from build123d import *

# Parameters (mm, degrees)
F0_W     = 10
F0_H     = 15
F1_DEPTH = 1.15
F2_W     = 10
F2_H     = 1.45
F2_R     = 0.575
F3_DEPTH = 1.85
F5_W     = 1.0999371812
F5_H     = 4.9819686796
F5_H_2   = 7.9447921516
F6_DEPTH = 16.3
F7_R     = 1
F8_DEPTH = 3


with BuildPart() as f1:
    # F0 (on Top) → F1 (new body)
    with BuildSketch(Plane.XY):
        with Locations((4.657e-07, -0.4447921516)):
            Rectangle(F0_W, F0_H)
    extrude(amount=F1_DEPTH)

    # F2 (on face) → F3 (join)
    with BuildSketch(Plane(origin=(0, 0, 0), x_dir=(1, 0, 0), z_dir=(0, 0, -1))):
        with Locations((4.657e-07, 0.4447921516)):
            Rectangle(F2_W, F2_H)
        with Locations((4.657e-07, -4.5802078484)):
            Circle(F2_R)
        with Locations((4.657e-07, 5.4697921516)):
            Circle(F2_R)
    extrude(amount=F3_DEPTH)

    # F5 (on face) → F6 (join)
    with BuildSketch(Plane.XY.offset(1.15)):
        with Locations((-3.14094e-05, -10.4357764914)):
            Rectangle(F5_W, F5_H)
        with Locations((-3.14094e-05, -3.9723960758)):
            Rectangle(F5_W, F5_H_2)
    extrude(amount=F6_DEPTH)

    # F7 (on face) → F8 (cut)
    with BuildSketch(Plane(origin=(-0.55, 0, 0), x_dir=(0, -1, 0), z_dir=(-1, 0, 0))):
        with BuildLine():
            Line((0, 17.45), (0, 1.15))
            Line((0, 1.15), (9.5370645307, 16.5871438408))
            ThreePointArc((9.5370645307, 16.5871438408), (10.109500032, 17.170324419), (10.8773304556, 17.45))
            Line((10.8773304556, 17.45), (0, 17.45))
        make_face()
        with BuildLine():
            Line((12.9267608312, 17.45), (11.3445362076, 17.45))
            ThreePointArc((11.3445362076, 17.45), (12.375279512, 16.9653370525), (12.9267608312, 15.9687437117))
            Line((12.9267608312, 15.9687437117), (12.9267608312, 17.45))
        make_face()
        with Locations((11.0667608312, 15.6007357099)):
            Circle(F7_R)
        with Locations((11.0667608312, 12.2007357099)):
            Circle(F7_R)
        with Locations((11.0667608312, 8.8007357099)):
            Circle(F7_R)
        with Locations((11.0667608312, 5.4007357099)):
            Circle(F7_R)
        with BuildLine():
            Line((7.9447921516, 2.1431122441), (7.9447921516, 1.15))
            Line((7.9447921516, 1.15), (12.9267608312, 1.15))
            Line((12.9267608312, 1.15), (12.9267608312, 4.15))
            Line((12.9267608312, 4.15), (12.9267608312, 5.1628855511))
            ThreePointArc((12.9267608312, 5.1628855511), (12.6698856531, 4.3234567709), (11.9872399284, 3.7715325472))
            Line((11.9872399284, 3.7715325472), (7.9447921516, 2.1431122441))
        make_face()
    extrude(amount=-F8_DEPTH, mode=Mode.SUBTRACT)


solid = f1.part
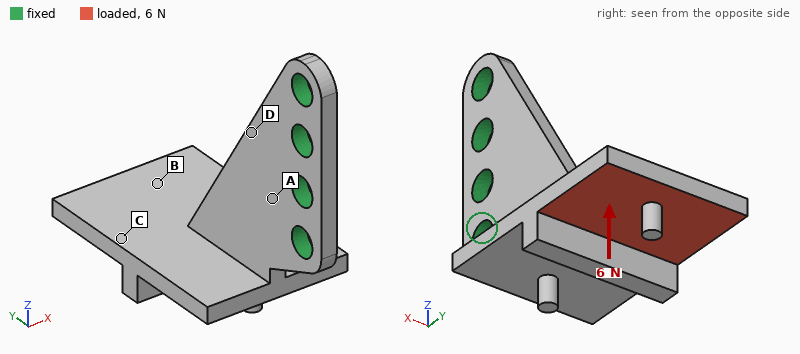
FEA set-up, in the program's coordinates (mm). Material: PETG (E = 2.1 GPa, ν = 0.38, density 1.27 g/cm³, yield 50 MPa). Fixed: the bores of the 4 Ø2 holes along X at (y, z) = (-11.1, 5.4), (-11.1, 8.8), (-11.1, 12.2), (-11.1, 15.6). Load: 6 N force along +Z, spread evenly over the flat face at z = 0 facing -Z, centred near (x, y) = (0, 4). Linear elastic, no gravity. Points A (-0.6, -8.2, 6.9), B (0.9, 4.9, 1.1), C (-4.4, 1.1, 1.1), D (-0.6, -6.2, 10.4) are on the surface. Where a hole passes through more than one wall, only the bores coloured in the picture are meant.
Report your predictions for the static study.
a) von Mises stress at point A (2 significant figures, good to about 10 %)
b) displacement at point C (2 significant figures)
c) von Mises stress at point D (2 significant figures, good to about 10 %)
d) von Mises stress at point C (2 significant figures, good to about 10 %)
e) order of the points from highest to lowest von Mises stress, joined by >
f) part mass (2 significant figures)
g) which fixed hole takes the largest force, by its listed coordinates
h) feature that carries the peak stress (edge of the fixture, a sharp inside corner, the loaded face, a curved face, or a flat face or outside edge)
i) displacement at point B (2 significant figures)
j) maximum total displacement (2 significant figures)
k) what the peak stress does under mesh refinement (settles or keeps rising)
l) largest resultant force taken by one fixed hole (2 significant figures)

2.2 MPa
0.11 mm
3.7 MPa
5.3 MPa
C > D > A > B
0.40 g
(-11.1, 5.4)
a sharp inside corner
0.24 mm
0.34 mm
keeps rising
12 N
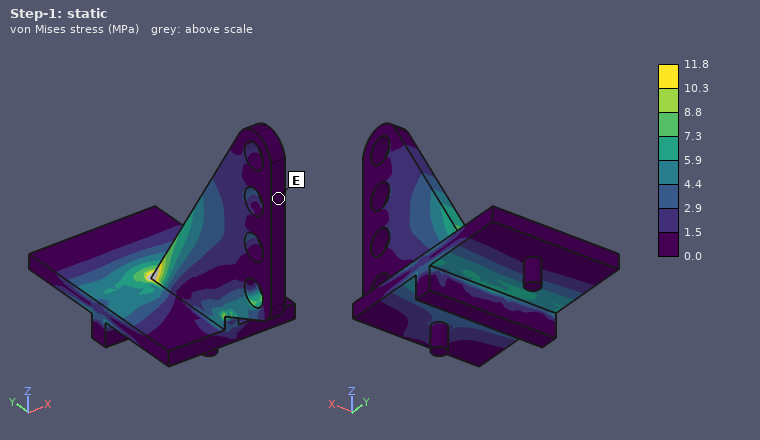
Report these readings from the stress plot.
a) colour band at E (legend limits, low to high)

0.0 to 1.5 MPa
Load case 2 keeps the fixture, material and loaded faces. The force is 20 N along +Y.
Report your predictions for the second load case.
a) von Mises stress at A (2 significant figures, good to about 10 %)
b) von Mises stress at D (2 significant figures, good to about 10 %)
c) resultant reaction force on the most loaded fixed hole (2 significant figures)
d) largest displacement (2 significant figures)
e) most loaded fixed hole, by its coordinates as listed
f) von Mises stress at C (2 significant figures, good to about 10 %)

2.0 MPa
5.3 MPa
34 N
0.29 mm
(-11.1, 5.4)
2.7 MPa
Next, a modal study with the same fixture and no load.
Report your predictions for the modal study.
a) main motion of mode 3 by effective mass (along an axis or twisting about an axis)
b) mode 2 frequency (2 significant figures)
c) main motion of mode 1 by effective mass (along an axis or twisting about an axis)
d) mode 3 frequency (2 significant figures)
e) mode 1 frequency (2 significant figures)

along Z
1700 Hz
along X
2300 Hz
530 Hz
